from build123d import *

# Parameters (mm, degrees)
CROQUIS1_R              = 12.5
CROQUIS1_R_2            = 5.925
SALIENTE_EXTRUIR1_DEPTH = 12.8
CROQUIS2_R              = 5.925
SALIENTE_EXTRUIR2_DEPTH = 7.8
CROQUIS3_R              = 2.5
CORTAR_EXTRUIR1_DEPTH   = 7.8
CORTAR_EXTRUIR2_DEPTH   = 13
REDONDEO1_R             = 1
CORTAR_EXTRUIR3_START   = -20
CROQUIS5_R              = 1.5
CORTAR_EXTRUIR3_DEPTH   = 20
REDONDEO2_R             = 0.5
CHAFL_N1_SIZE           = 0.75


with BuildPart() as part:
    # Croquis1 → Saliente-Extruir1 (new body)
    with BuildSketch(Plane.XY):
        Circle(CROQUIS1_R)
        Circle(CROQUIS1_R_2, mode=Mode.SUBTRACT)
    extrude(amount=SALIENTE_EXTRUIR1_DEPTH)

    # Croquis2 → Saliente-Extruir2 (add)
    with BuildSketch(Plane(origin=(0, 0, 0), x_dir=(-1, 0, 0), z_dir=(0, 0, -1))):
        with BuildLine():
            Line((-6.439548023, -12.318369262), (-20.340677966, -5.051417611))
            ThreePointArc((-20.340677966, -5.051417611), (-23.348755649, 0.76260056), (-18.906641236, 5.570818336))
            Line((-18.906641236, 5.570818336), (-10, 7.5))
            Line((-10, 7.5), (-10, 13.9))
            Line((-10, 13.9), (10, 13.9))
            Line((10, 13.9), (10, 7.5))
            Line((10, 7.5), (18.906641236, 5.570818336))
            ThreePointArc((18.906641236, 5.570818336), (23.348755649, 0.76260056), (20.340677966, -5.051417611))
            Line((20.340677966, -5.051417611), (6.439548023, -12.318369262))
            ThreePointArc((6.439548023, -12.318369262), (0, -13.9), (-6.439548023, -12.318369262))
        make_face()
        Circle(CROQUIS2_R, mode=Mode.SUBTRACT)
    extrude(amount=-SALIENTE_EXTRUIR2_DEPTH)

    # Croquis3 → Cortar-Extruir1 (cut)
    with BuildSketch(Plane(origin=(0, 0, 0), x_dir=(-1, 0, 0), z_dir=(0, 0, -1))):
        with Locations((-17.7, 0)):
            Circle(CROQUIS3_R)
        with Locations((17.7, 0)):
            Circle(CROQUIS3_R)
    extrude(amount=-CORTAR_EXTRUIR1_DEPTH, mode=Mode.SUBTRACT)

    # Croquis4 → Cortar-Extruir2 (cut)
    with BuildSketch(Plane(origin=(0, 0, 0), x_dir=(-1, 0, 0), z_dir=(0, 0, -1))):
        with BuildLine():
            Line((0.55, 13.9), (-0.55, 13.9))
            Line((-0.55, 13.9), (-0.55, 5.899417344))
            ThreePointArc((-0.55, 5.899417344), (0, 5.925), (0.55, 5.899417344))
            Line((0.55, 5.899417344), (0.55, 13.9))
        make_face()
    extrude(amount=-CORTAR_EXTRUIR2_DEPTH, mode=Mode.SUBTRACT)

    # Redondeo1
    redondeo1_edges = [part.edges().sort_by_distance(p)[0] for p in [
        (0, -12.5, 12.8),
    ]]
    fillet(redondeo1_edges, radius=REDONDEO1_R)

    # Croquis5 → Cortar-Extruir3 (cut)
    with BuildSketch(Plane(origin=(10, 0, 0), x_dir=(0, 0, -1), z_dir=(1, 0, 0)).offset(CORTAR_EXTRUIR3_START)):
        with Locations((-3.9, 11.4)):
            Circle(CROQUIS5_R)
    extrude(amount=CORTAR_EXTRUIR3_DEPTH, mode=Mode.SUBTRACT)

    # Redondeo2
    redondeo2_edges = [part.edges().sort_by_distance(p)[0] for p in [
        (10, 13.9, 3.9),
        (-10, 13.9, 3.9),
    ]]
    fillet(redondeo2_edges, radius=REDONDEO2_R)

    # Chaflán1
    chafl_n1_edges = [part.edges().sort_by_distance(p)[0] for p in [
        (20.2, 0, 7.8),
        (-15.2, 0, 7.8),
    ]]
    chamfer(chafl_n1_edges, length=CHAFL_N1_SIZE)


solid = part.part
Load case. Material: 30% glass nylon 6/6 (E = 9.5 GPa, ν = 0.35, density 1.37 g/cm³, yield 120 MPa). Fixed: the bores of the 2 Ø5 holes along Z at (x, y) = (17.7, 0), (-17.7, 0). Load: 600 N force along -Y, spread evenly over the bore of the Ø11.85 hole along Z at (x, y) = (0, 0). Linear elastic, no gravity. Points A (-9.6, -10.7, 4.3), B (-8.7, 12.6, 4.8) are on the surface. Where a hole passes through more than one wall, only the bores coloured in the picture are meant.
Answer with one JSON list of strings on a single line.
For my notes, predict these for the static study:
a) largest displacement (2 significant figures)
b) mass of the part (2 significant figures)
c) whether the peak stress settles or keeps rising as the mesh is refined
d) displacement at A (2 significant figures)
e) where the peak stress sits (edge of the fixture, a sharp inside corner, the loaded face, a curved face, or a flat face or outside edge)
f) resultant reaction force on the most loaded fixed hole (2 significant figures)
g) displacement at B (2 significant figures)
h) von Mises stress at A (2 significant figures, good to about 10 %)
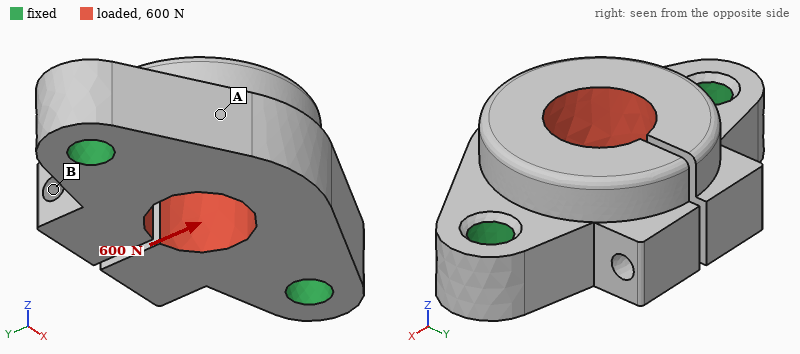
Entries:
["45 µm", "9.9 g", "keeps rising", "15 µm", "edge of the fixture", "390 N", "28 µm", "7.0 MPa"]
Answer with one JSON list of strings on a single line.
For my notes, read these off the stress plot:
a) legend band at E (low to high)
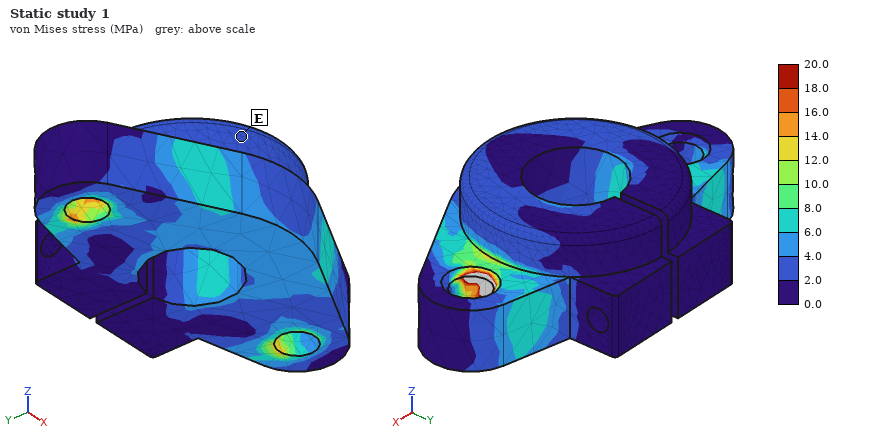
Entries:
["2.0 to 4.0 MPa"]
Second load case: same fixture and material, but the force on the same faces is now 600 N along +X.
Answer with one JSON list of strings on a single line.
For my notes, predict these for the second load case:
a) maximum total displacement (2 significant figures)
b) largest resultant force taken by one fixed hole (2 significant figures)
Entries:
["13 µm", "300 N"]
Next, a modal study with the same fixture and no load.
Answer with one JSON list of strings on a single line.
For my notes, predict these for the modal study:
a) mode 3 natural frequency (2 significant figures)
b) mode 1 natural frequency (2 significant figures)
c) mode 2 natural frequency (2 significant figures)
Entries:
["8600 Hz", "7800 Hz", "8500 Hz"]
